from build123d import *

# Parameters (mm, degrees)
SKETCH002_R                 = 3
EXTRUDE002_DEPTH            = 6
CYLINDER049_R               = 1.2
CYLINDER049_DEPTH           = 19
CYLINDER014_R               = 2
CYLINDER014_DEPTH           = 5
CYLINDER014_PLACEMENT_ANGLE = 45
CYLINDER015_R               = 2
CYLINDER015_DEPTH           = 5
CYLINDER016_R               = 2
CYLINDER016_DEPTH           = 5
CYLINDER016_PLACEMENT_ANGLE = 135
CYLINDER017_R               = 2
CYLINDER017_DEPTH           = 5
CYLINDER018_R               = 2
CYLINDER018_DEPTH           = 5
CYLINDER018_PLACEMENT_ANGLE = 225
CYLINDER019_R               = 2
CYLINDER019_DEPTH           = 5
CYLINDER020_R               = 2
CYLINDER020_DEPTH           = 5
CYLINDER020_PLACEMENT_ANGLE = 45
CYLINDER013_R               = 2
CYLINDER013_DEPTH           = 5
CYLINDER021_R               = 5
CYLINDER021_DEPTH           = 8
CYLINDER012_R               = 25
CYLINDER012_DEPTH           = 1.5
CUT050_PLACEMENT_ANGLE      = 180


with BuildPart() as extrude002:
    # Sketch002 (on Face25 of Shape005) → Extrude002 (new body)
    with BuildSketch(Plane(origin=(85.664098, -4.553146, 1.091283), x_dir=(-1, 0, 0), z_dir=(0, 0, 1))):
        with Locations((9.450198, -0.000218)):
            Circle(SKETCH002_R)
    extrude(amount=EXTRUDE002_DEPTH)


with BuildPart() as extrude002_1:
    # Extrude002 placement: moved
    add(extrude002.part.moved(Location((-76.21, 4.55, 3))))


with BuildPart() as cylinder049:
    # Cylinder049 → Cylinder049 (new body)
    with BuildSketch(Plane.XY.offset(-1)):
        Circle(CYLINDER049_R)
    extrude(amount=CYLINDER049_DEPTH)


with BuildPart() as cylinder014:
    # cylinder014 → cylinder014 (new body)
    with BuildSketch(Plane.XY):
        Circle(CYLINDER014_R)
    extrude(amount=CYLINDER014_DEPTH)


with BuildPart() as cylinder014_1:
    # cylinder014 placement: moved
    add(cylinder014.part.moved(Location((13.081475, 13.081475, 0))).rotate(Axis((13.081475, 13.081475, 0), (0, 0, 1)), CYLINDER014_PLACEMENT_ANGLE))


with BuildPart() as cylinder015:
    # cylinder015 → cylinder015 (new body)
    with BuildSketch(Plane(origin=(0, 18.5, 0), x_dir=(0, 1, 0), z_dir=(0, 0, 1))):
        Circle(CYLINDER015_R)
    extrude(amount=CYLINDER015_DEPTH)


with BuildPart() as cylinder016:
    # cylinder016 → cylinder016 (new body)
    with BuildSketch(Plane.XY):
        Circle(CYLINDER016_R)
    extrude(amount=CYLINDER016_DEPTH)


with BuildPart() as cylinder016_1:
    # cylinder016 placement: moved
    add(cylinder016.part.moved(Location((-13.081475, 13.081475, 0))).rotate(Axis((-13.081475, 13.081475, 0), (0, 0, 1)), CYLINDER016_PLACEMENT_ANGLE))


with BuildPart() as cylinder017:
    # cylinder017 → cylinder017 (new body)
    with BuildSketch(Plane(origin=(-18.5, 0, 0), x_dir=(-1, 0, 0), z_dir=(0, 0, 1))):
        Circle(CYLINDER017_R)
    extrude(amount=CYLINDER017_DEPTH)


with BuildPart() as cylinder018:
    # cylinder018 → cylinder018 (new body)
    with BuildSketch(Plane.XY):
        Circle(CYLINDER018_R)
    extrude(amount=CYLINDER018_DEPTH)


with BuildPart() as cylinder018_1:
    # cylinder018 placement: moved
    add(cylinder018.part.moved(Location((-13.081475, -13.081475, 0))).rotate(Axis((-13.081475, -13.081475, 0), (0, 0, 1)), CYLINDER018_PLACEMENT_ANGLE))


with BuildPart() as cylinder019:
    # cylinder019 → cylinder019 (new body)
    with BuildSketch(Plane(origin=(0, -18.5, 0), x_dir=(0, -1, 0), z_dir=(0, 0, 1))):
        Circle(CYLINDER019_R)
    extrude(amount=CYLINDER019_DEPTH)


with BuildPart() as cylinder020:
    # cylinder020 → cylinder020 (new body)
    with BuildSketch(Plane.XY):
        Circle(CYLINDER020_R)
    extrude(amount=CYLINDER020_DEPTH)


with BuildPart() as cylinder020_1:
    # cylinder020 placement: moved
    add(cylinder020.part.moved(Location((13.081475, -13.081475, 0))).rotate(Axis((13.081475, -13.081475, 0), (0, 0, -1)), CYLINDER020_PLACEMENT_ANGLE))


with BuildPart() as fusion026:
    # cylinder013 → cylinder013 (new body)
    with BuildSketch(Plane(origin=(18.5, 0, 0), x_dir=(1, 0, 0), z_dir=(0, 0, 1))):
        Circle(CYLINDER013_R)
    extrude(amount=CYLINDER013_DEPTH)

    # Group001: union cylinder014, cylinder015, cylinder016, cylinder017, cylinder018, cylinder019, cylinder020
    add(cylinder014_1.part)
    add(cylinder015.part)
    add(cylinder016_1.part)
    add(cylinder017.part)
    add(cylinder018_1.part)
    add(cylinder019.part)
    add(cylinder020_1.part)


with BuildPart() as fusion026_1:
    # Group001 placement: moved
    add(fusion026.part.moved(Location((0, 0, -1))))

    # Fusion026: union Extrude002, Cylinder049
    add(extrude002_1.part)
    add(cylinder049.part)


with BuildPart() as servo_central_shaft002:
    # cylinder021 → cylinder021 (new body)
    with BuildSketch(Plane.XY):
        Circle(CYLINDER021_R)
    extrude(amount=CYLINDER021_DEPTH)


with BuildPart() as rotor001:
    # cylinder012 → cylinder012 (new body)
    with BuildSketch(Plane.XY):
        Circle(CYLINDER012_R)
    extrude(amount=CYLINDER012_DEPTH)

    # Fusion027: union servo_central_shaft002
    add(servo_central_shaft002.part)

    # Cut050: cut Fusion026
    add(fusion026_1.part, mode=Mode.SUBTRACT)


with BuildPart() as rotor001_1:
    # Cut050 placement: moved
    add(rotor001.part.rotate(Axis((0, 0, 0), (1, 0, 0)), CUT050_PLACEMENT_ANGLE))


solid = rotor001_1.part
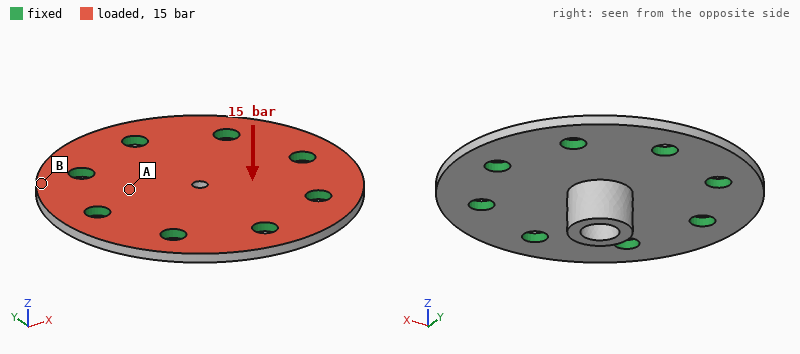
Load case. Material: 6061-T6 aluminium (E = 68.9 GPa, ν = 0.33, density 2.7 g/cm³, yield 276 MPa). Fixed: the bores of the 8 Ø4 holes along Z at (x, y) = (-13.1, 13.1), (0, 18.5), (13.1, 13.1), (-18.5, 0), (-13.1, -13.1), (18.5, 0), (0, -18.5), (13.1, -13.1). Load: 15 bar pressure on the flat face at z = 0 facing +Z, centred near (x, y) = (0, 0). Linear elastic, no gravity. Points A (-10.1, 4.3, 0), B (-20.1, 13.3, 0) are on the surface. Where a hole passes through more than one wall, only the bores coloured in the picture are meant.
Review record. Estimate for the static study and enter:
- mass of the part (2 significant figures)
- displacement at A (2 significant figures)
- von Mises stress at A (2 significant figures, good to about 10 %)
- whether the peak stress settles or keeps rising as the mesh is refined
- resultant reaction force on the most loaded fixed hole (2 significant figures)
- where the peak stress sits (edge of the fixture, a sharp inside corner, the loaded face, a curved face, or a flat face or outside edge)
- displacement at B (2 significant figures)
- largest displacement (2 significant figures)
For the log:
8.6 g
37 µm
44 MPa
keeps rising
350 N
edge of the fixture
11 µm
70 µm
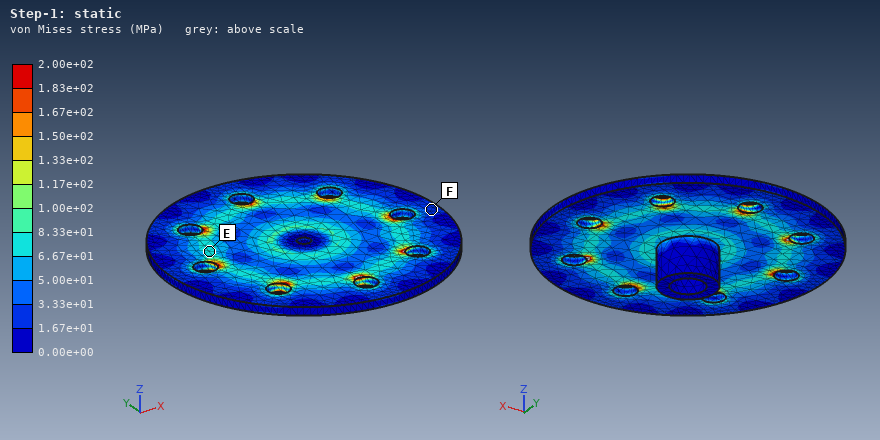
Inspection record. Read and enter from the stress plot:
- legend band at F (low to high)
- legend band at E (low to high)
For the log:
1.67e+01 to 3.33e+01 MPa
6.67e+01 to 8.33e+01 MPa
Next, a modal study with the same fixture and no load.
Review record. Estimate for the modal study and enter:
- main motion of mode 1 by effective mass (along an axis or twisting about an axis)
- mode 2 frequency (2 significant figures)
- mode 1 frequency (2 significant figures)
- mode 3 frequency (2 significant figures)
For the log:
along Z
17 kHz
9600 Hz
17 kHz
